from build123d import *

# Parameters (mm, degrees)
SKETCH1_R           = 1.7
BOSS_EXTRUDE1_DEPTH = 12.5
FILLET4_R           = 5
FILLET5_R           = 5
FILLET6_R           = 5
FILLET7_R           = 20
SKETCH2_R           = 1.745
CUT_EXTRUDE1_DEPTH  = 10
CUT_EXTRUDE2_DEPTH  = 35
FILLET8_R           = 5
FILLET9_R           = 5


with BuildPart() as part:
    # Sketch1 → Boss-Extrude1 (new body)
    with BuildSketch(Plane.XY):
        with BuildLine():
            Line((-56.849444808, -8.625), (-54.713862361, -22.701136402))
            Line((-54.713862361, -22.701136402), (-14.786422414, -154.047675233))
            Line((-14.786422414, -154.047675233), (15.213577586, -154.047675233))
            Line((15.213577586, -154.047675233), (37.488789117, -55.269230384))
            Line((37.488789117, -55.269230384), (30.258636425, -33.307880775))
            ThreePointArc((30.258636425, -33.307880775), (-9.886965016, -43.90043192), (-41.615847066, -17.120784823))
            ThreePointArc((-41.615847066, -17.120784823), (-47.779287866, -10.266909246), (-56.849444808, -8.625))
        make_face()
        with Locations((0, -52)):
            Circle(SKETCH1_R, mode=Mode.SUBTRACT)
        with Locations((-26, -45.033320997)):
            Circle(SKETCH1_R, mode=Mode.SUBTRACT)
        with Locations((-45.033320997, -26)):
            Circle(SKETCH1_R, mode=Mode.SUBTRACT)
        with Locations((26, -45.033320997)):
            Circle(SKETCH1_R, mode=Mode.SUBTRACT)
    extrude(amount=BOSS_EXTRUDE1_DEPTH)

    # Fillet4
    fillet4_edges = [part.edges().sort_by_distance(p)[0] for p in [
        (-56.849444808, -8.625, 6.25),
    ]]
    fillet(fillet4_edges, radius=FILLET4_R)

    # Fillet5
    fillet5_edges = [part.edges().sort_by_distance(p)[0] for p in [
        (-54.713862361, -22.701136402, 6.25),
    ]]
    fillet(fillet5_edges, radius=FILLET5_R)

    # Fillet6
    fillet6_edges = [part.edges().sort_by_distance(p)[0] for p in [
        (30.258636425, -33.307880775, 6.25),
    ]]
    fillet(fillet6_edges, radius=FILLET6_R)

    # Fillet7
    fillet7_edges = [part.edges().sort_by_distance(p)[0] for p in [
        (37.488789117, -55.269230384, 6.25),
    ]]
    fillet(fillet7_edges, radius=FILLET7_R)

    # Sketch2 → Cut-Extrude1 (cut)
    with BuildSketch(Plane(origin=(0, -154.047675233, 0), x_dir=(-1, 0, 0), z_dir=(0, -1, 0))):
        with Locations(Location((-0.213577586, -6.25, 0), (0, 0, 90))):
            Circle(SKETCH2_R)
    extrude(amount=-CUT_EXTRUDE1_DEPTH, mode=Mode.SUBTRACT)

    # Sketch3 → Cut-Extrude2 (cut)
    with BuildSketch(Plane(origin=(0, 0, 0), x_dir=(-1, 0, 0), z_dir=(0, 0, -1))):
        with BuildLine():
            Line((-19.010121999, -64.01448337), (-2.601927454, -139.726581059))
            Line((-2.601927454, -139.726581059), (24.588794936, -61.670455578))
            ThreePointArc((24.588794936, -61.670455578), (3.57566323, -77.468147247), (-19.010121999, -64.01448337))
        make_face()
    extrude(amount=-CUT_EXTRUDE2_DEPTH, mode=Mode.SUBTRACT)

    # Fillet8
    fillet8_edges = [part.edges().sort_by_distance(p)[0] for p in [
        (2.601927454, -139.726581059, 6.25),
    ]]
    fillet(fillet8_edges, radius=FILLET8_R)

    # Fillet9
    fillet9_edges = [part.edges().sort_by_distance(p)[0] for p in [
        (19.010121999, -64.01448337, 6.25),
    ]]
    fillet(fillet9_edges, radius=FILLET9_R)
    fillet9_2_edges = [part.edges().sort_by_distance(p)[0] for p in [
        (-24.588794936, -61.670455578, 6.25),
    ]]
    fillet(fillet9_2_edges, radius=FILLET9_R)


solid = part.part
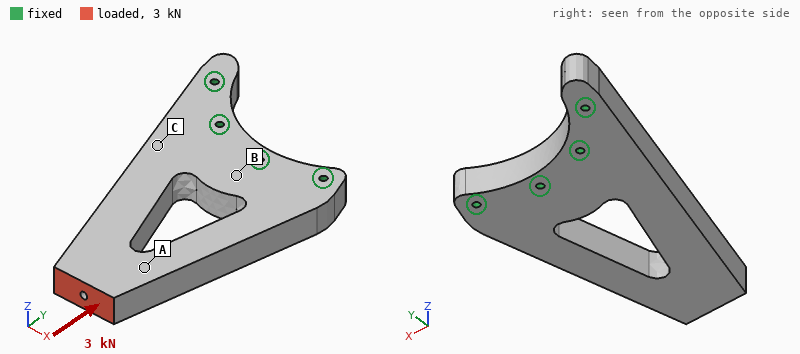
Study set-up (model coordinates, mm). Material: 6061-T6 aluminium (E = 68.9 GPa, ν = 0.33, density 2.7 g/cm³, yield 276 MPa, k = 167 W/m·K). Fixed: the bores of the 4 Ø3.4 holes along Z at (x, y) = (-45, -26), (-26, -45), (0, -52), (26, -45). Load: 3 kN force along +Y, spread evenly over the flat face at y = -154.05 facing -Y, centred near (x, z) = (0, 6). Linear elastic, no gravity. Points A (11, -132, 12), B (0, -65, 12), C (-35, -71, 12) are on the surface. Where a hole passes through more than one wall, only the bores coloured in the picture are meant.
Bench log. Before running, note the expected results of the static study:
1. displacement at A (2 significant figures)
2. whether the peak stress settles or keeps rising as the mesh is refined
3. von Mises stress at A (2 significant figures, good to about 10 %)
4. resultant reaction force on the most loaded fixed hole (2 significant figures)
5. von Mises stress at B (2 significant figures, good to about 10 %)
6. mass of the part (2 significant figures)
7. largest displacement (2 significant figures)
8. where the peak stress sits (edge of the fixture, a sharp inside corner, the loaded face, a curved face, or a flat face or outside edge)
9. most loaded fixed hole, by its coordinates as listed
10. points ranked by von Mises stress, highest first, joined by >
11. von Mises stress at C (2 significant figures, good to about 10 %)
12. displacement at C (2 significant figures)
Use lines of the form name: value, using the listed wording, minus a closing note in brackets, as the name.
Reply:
displacement at A: 10 µm
whether the peak stress settles or keeps rising as the mesh is refined: keeps rising
von Mises stress at A: 8.2 MPa
resultant reaction force on the most loaded fixed hole: 1.3 kN
von Mises stress at B: 1.8 MPa
mass of the part: 210 g
largest displacement: 13 µm
where the peak stress sits: edge of the fixture
most loaded fixed hole, by its coordinates as listed: (26, -45)
points ranked by von Mises stress, highest first, joined by >: A > C > B
von Mises stress at C: 4.2 MPa
displacement at C: 1.9 µm
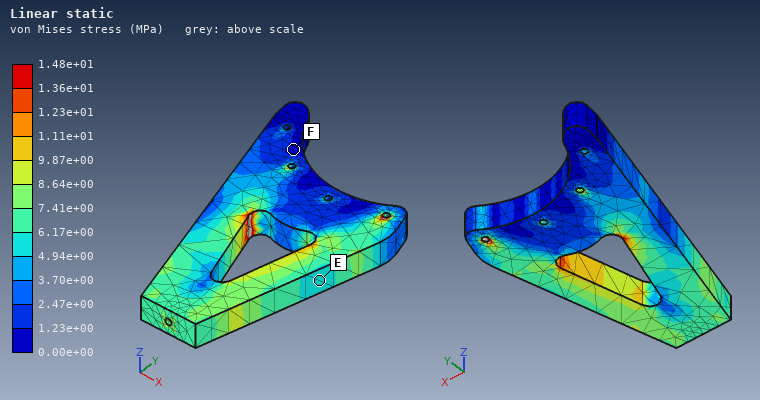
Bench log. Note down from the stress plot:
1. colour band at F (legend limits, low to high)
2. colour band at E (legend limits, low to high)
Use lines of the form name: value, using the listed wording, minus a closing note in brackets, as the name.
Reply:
colour band at F: 0.00e+00 to 1.23e+00 MPa
colour band at E: 4.94e+00 to 6.17e+00 MPa
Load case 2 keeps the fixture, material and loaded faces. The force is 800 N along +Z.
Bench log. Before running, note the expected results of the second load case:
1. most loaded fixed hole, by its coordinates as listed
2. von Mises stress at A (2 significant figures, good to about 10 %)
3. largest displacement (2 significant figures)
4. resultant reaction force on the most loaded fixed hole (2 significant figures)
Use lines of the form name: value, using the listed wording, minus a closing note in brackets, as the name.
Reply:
most loaded fixed hole, by its coordinates as listed: (0, -52)
von Mises stress at A: 19 MPa
largest displacement: 0.65 mm
resultant reaction force on the most loaded fixed hole: 1.5 kN
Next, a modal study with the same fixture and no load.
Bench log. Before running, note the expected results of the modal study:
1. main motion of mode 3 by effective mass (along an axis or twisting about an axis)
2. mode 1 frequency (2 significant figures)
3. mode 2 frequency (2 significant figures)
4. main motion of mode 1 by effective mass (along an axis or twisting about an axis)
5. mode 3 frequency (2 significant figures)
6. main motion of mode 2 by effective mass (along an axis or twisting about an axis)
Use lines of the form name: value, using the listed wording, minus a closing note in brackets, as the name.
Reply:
main motion of mode 3 by effective mass: along X
mode 1 frequency: 1000 Hz
mode 2 frequency: 3800 Hz
main motion of mode 1 by effective mass: along Z
mode 3 frequency: 4000 Hz
main motion of mode 2 by effective mass: twisting about Y
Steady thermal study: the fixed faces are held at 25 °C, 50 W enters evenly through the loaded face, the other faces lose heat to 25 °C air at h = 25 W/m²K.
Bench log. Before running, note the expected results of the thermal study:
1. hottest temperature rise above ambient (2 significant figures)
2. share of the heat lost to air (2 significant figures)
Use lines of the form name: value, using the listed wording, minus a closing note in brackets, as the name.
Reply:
hottest temperature rise above ambient: 60 K
share of the heat lost to air: 17 %
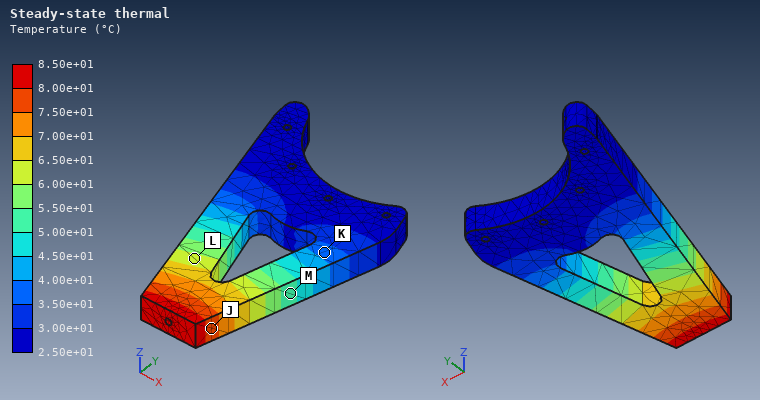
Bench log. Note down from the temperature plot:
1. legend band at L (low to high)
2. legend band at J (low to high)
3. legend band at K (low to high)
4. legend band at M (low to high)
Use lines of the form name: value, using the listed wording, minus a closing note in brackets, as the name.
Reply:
legend band at L: 6.00e+01 to 6.50e+01 °C
legend band at J: 7.50e+01 to 8.00e+01 °C
legend band at K: 3.50e+01 to 4.00e+01 °C
legend band at M: 5.00e+01 to 5.50e+01 °C
